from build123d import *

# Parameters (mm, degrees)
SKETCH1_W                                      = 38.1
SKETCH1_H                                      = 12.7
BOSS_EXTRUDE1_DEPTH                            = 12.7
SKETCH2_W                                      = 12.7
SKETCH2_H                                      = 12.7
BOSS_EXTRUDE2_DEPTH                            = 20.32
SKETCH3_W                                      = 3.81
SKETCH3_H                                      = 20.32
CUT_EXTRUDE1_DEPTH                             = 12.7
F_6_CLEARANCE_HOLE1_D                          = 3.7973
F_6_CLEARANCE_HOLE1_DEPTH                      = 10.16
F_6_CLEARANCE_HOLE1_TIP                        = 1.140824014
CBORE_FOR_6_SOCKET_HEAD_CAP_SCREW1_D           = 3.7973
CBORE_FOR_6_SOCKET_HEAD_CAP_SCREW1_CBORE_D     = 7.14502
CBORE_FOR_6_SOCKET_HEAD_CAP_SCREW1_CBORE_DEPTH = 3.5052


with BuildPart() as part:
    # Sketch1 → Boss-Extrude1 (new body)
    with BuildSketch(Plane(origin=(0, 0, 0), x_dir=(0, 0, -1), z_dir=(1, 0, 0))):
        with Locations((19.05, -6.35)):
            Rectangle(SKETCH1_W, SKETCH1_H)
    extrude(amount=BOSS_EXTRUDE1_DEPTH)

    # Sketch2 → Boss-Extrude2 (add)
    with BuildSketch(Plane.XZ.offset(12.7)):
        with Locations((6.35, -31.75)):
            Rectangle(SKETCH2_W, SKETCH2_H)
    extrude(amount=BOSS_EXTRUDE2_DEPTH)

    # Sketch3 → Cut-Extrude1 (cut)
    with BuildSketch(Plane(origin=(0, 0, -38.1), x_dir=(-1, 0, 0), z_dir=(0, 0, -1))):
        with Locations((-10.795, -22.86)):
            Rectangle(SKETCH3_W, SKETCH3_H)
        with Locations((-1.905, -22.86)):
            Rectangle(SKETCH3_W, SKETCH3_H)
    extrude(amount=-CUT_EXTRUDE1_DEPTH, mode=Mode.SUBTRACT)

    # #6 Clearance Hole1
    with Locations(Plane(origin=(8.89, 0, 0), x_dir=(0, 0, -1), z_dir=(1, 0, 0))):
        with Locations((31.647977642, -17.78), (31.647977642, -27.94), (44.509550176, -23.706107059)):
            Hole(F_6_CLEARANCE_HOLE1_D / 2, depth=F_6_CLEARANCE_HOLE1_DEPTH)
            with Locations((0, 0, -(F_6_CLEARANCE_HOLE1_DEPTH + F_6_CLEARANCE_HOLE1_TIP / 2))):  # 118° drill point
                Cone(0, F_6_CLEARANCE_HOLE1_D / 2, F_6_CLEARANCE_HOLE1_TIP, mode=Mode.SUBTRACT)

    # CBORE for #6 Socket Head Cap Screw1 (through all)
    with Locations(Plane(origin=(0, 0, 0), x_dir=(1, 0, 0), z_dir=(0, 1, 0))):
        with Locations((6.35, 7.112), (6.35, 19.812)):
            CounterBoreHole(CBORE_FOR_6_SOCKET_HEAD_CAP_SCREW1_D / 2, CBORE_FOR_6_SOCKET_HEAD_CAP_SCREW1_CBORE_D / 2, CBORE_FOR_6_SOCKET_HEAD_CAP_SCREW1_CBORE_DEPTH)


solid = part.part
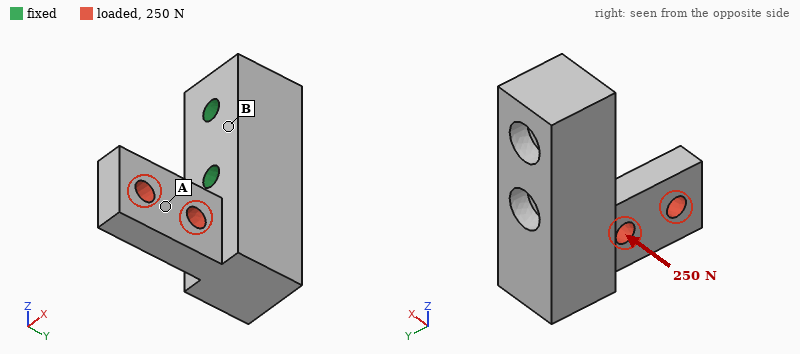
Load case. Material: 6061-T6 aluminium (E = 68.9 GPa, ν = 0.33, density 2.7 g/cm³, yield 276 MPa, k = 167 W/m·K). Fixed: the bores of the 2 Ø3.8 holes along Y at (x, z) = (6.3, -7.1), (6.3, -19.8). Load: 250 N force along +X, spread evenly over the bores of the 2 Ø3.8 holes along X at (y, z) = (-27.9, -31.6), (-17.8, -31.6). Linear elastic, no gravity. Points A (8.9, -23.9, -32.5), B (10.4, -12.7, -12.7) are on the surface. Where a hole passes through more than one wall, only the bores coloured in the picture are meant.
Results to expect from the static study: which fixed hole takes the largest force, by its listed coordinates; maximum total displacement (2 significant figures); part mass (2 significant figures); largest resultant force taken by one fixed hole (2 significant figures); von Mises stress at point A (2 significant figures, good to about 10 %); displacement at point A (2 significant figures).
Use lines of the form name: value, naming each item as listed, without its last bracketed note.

which fixed hole takes the largest force, by its listed coordinates: (6.3, -19.8)
maximum total displacement: 59 µm
part mass: 18 g
largest resultant force taken by one fixed hole: 380 N
von Mises stress at point A: 9.9 MPa
displacement at point A: 31 µm
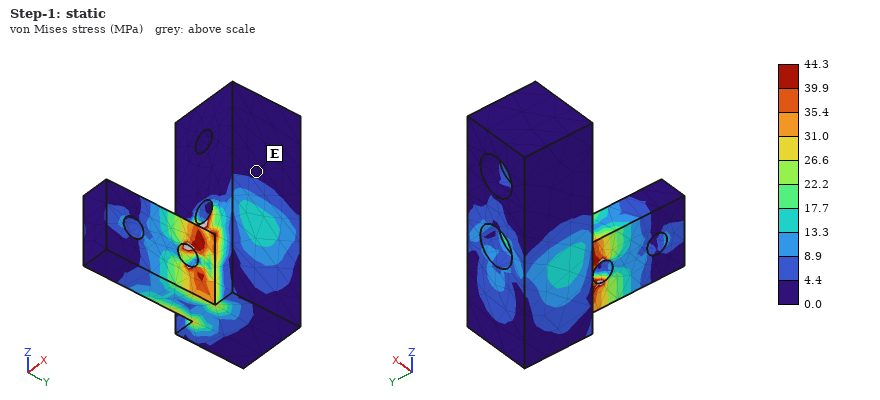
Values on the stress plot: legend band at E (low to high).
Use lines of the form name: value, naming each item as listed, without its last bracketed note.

legend band at E: 0.0 to 4.4 MPa
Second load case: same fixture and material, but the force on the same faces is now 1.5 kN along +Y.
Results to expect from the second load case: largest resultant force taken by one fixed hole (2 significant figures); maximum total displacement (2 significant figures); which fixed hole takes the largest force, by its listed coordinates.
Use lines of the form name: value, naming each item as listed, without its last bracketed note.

largest resultant force taken by one fixed hole: 1.9 kN
maximum total displacement: 44 µm
which fixed hole takes the largest force, by its listed coordinates: (6.3, -19.8)
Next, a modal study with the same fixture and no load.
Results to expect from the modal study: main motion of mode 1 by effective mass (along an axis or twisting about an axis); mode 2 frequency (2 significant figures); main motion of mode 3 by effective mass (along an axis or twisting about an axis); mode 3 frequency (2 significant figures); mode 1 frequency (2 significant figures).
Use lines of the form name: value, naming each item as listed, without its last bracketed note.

main motion of mode 1 by effective mass: along X
mode 2 frequency: 10 kHz
main motion of mode 3 by effective mass: along X
mode 3 frequency: 17 kHz
mode 1 frequency: 7100 Hz
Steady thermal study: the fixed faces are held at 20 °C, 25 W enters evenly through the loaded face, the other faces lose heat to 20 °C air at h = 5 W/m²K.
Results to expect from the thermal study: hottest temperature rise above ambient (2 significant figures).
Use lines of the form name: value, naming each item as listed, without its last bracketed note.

hottest temperature rise above ambient: 44 K
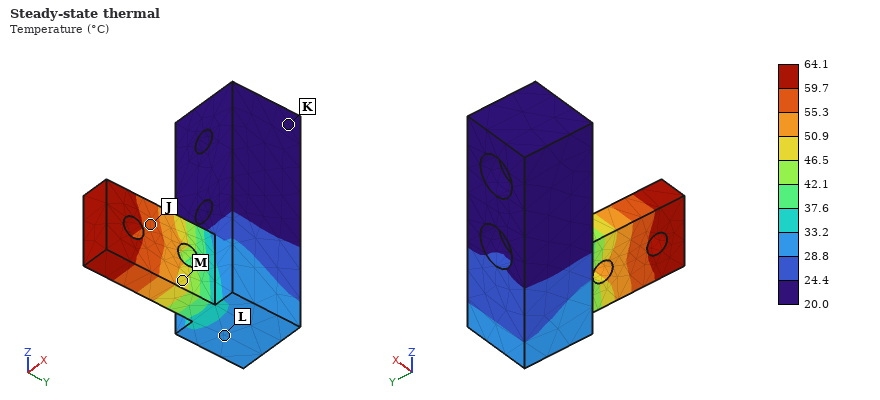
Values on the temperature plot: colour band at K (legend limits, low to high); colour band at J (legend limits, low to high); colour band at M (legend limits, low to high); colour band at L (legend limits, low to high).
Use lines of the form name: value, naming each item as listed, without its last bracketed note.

colour band at K: 20.0 to 24.4 °C
colour band at J: 55.3 to 59.7 °C
colour band at M: 46.5 to 50.9 °C
colour band at L: 28.8 to 33.2 °C
